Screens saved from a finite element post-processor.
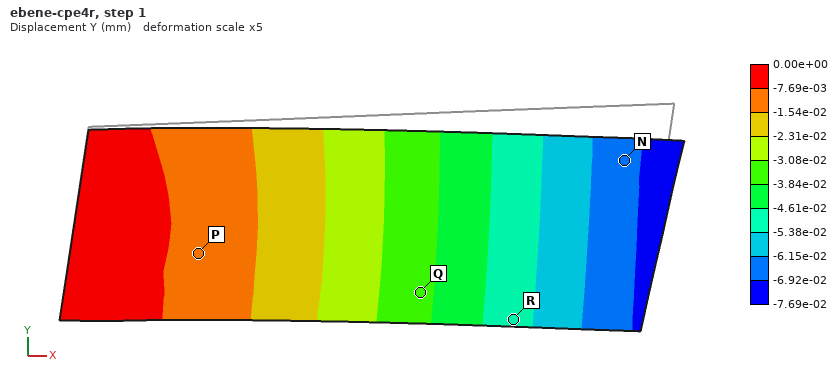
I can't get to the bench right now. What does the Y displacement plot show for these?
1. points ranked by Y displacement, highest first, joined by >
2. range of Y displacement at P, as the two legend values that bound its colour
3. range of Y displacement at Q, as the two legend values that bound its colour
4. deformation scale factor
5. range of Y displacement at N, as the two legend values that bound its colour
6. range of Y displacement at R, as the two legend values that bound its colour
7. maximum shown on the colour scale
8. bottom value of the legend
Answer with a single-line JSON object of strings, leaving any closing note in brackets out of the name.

{"points ranked by Y displacement, highest first, joined by >": "P > Q > R > N", "range of Y displacement at P, as the two legend values that bound its colour": "-1.54e-02 to -7.69e-03 mm", "range of Y displacement at Q, as the two legend values that bound its colour": "-3.84e-02 to -3.08e-02 mm", "deformation scale factor": "5", "range of Y displacement at N, as the two legend values that bound its colour": "-6.92e-02 to -6.15e-02 mm", "range of Y displacement at R, as the two legend values that bound its colour": "-5.38e-02 to -4.61e-02 mm", "maximum shown on the colour scale": "0.00e+00 mm", "bottom value of the legend": "-7.69e-02 mm"}
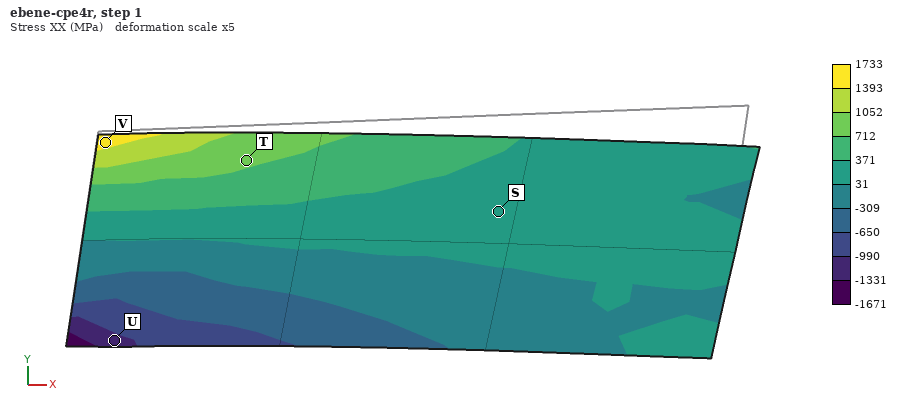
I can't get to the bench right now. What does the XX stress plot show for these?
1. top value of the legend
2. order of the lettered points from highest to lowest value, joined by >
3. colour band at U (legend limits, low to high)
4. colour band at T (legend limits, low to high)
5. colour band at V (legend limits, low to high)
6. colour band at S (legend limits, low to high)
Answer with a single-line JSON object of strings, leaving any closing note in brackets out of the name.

{"top value of the legend": "1733 MPa", "order of the lettered points from highest to lowest value, joined by >": "V > T > S > U", "colour band at U": "-1331 to -990 MPa", "colour band at T": "712 to 1052 MPa", "colour band at V": "1393 to 1733 MPa", "colour band at S": "31 to 371 MPa"}
